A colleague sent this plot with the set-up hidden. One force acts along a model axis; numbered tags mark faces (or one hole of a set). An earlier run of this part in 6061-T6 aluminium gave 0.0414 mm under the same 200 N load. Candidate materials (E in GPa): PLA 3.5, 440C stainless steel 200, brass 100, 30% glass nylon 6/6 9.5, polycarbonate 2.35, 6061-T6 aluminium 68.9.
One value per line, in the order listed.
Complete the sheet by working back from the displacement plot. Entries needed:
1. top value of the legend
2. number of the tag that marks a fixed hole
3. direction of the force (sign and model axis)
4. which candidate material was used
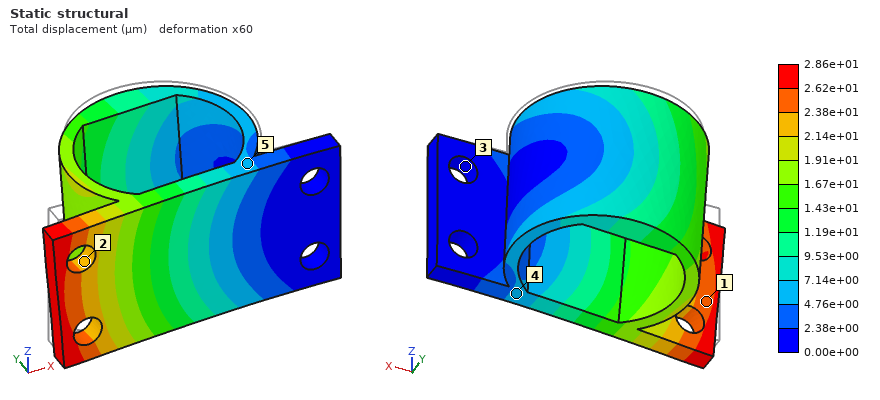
2.86e+01 µm
3
-Z
brass
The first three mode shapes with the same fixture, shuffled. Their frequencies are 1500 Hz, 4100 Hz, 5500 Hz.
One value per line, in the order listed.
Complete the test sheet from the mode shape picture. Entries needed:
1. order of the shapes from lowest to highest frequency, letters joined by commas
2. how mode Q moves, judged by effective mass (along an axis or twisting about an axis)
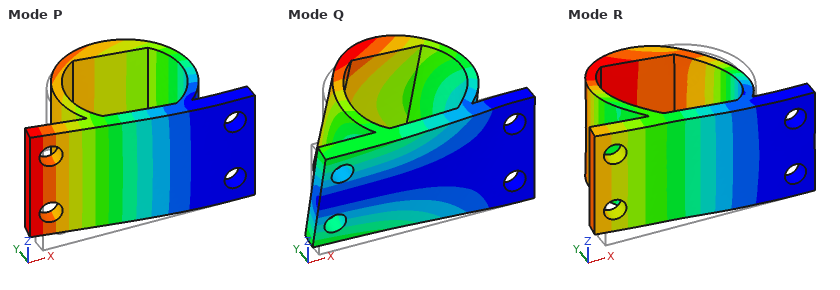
P, Q, R
along Z
